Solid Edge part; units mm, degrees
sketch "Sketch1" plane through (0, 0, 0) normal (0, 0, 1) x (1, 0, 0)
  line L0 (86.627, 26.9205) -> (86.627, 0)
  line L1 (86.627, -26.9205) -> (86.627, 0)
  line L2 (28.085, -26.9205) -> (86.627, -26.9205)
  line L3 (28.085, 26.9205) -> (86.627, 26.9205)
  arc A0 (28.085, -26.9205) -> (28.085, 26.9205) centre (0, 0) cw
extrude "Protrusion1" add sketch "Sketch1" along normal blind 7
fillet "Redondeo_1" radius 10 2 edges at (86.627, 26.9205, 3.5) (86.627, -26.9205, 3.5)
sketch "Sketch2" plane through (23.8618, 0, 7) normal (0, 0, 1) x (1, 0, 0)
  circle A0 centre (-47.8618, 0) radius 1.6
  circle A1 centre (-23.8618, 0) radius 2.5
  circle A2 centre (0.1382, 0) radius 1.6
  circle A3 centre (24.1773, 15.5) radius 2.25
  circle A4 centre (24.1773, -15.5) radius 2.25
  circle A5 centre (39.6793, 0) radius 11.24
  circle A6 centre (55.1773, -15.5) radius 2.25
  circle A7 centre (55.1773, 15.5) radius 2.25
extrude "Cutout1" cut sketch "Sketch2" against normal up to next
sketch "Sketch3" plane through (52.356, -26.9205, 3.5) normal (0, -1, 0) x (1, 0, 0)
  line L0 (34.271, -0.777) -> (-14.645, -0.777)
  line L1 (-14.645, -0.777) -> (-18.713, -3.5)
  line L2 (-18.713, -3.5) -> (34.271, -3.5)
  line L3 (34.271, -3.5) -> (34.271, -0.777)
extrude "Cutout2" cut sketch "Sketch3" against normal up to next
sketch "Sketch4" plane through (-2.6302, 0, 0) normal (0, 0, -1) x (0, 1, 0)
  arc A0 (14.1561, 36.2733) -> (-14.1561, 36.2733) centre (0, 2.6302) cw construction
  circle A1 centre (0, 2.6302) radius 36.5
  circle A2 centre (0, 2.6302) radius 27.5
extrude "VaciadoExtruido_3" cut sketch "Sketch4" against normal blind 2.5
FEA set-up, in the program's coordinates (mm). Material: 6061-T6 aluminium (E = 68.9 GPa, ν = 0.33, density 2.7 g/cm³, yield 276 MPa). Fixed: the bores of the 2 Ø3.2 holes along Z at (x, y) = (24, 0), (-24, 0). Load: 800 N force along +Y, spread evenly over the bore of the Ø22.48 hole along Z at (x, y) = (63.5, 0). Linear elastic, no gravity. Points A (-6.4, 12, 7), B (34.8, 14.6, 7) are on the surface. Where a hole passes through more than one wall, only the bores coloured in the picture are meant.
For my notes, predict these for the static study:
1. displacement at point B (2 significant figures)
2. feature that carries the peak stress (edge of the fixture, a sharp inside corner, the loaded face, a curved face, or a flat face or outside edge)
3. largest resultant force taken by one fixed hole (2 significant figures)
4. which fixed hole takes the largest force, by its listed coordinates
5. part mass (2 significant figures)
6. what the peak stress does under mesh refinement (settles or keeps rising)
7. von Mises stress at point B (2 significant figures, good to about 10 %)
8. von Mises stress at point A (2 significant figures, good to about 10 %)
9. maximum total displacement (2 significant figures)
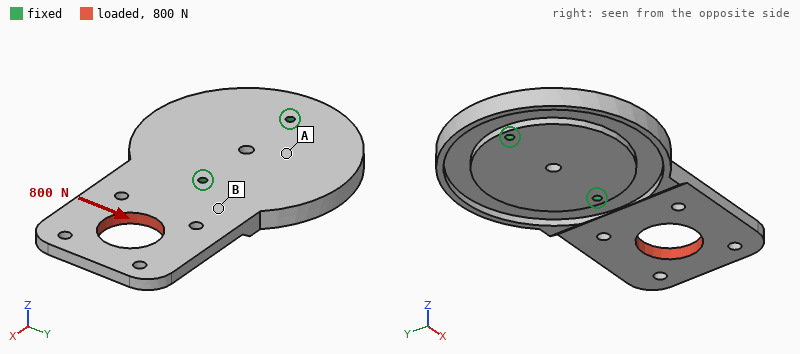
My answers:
6.0 µm
edge of the fixture
1.4 kN
(24, 0)
100 g
keeps rising
5.6 MPa
2.9 MPa
32 µm
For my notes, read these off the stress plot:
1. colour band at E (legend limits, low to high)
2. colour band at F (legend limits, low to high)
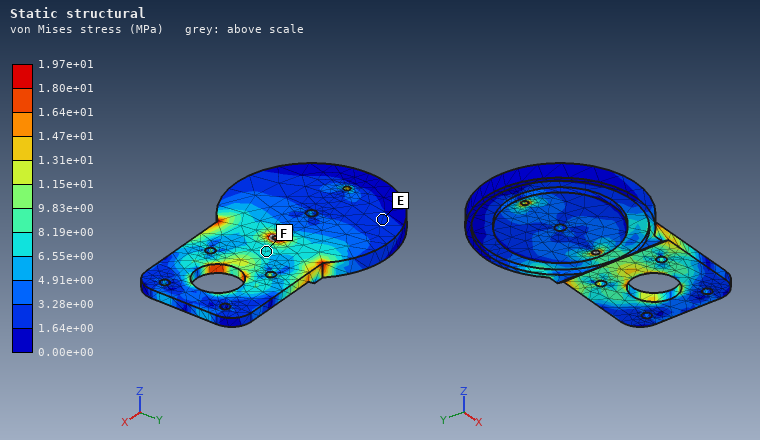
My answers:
1.64e+00 to 3.28e+00 MPa
6.55e+00 to 8.19e+00 MPa
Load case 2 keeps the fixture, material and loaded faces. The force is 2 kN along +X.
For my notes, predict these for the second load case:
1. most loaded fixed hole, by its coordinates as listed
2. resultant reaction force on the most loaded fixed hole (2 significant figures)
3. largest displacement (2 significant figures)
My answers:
(24, 0)
1.4 kN
23 µm
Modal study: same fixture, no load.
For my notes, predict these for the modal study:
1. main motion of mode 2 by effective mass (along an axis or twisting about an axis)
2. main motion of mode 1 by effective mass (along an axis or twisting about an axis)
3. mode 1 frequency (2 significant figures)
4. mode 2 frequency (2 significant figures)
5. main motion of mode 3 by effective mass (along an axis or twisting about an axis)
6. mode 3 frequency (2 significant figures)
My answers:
twisting about X
along Z
1000 Hz
2100 Hz
twisting about X
3300 Hz
